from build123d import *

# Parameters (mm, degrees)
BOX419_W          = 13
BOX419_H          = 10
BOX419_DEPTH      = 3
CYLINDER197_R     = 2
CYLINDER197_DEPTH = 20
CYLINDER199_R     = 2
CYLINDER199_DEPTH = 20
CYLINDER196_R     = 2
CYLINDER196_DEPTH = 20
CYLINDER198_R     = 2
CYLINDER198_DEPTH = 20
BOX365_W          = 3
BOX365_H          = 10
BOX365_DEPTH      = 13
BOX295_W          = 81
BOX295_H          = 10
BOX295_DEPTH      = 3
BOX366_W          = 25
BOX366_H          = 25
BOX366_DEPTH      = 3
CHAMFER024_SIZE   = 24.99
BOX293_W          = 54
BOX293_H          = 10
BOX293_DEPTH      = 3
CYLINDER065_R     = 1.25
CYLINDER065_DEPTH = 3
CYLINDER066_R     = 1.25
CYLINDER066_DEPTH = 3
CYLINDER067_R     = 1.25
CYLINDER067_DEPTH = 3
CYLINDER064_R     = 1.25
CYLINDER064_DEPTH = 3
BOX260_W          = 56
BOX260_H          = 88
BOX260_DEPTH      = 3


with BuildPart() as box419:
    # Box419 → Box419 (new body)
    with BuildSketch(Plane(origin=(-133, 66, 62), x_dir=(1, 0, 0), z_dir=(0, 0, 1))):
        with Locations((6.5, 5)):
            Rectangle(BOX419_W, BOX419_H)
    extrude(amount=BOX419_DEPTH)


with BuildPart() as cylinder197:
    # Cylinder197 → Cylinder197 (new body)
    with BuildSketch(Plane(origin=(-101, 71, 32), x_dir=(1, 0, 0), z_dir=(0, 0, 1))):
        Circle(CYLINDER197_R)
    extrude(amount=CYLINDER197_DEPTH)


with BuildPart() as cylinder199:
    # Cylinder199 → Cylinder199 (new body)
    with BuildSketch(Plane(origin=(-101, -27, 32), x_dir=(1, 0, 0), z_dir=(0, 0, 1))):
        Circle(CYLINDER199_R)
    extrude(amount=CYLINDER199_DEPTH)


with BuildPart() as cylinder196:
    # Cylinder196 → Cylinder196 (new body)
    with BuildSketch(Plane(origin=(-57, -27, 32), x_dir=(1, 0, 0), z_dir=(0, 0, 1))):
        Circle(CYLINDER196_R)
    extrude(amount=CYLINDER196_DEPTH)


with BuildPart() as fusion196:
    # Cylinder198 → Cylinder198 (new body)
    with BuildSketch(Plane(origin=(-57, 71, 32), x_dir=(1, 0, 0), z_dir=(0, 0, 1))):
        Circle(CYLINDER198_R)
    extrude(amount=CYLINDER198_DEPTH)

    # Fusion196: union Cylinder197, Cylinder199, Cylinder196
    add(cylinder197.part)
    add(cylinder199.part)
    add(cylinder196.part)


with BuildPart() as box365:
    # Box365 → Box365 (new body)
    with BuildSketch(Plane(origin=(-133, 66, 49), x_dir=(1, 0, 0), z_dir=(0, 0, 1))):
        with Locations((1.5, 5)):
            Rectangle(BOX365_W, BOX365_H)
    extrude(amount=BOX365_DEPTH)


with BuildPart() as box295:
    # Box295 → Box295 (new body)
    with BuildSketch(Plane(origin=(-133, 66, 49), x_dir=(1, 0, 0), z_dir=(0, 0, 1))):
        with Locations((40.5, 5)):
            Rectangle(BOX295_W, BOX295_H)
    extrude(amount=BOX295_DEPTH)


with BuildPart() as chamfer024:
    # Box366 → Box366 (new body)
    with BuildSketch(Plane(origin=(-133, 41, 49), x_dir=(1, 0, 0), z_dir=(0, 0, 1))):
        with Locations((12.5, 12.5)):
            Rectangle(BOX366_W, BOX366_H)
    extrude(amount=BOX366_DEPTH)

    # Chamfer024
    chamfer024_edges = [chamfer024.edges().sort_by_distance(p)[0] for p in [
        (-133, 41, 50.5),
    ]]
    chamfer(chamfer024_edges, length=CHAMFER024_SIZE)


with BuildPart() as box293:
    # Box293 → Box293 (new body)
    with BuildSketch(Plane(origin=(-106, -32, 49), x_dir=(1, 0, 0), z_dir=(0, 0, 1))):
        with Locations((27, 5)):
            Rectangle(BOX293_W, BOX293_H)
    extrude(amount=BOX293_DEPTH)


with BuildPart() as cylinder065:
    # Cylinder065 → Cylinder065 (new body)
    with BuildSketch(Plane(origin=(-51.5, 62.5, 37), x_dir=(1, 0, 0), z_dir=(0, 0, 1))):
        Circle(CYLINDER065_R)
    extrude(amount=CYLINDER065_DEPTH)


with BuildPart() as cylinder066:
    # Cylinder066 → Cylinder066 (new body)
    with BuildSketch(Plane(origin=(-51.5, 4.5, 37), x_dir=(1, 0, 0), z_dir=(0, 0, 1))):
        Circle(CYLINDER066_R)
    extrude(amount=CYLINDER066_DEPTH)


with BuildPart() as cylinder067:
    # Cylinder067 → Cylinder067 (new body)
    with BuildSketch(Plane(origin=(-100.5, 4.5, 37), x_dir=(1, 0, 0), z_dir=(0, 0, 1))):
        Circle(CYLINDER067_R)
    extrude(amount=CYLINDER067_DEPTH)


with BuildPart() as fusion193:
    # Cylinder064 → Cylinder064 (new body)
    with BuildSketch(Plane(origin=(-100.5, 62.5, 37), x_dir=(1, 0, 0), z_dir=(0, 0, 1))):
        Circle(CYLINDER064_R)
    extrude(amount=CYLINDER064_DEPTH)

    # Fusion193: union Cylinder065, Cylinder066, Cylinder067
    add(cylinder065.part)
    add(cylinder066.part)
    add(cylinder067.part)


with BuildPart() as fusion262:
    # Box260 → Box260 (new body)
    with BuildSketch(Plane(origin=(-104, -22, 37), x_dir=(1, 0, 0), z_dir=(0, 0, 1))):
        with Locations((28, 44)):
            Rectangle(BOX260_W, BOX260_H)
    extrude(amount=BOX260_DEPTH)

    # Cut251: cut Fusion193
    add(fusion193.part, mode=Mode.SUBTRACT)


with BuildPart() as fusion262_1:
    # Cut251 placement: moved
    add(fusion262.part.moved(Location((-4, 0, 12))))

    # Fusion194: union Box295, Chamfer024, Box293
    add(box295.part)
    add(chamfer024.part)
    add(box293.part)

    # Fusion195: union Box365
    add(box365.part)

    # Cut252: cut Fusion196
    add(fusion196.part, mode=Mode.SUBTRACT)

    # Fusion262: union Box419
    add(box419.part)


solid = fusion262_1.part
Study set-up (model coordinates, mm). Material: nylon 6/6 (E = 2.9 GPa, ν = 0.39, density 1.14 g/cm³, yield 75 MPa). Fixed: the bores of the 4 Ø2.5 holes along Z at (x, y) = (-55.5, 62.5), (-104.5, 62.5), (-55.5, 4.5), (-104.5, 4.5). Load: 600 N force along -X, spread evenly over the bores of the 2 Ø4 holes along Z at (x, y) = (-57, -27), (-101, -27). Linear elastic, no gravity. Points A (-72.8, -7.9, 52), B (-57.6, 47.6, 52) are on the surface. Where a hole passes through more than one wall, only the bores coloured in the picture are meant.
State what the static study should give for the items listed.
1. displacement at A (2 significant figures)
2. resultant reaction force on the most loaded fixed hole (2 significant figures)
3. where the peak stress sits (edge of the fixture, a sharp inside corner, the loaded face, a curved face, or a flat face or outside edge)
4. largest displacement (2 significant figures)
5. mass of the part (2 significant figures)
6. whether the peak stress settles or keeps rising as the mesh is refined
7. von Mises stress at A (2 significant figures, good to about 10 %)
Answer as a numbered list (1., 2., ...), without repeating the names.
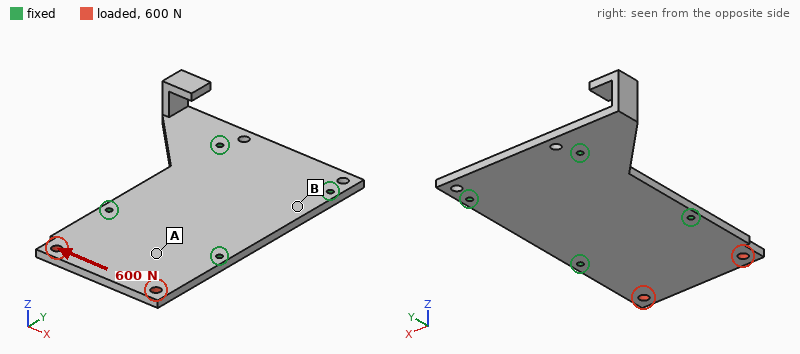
1. 0.080 mm
2. 470 N
3. edge of the fixture
4. 0.26 mm
5. 23 g
6. keeps rising
7. 7.8 MPa
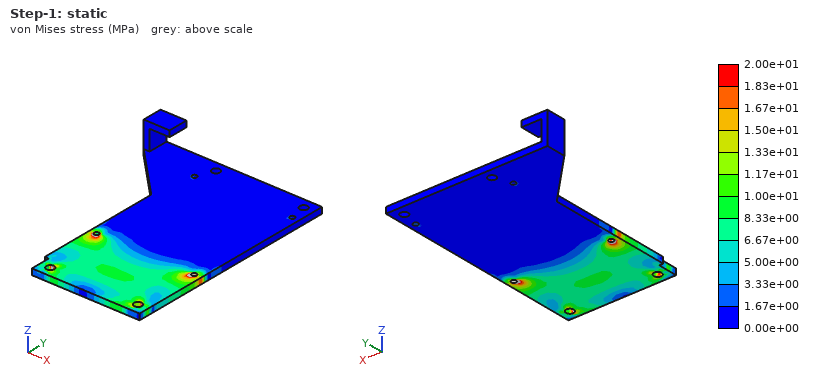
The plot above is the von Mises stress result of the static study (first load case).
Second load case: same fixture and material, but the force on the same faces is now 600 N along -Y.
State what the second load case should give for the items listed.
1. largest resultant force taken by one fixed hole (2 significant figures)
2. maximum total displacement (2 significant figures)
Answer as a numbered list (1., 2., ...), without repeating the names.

1. 260 N
2. 0.11 mm
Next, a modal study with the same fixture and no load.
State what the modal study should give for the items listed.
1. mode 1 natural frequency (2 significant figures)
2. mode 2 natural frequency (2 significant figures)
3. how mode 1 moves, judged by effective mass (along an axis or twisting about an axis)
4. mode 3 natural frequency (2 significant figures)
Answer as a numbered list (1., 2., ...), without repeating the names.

1. 480 Hz
2. 610 Hz
3. along Z
4. 1100 Hz
